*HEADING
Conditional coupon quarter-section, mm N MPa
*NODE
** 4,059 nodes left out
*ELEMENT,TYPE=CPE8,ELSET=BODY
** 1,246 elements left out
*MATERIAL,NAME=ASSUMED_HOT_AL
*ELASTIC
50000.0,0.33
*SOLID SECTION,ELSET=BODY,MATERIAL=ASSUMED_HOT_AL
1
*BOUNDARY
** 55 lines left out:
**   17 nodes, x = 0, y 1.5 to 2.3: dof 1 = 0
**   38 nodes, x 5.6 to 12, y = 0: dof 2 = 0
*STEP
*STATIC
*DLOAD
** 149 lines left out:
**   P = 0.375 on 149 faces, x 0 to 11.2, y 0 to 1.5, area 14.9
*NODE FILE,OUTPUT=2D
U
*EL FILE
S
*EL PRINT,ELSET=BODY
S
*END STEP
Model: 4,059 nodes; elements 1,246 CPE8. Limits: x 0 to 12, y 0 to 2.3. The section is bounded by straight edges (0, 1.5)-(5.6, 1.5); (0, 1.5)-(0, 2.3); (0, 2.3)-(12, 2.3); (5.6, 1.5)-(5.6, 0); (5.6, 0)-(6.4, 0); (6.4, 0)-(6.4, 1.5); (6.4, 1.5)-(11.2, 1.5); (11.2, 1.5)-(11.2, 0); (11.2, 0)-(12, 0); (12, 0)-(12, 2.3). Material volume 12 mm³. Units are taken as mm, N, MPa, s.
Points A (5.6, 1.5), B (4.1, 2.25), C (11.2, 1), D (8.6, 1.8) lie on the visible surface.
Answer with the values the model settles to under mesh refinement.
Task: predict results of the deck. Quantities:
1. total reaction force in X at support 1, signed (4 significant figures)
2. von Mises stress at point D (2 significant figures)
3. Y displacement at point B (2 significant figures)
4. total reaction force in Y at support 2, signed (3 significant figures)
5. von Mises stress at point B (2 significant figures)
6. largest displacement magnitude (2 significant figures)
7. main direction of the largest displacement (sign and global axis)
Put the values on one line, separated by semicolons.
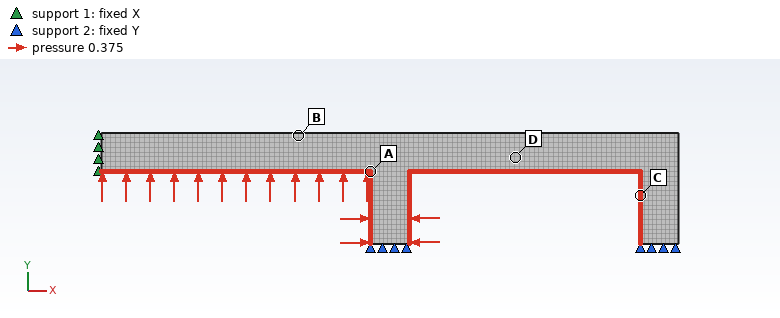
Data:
-0.5625 N; 1.9 MPa; 0.0040 mm; -3.90 N; 3.6 MPa; 0.011 mm; +Y
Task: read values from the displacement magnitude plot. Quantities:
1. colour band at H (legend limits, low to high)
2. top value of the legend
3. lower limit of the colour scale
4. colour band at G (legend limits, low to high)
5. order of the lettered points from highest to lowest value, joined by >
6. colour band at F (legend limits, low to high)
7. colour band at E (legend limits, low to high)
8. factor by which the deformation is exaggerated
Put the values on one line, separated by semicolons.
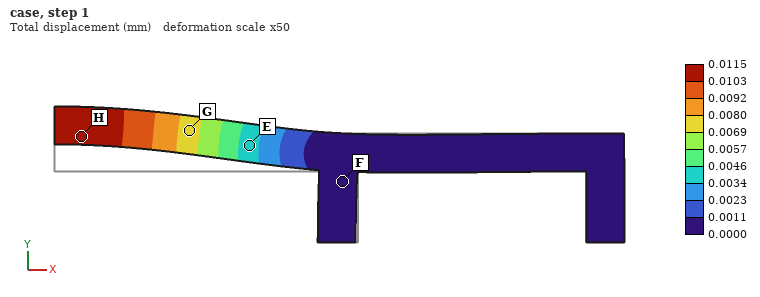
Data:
0.0103 to 0.0115 mm; 0.0115 mm; 0.0000 mm; 0.0069 to 0.0080 mm; H > G > E > F; 0.0000 to 0.0011 mm; 0.0034 to 0.0046 mm; 50
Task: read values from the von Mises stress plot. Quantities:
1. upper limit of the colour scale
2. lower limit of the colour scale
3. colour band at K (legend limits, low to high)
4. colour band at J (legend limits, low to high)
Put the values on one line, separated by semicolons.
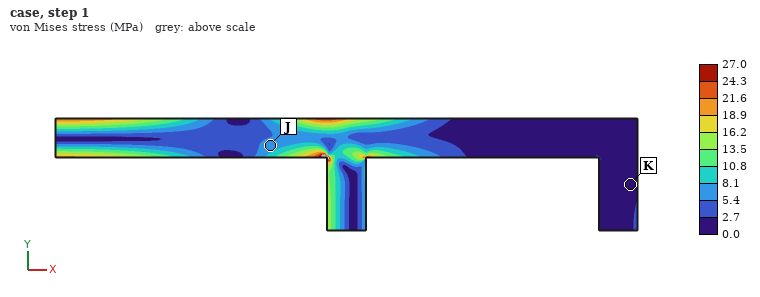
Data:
27.0 MPa; 0.0 MPa; 0.0 to 2.7 MPa; 5.4 to 8.1 MPa
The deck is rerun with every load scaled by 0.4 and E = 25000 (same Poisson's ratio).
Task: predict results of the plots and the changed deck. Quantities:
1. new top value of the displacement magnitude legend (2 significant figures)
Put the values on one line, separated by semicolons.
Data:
0.0092 mm
